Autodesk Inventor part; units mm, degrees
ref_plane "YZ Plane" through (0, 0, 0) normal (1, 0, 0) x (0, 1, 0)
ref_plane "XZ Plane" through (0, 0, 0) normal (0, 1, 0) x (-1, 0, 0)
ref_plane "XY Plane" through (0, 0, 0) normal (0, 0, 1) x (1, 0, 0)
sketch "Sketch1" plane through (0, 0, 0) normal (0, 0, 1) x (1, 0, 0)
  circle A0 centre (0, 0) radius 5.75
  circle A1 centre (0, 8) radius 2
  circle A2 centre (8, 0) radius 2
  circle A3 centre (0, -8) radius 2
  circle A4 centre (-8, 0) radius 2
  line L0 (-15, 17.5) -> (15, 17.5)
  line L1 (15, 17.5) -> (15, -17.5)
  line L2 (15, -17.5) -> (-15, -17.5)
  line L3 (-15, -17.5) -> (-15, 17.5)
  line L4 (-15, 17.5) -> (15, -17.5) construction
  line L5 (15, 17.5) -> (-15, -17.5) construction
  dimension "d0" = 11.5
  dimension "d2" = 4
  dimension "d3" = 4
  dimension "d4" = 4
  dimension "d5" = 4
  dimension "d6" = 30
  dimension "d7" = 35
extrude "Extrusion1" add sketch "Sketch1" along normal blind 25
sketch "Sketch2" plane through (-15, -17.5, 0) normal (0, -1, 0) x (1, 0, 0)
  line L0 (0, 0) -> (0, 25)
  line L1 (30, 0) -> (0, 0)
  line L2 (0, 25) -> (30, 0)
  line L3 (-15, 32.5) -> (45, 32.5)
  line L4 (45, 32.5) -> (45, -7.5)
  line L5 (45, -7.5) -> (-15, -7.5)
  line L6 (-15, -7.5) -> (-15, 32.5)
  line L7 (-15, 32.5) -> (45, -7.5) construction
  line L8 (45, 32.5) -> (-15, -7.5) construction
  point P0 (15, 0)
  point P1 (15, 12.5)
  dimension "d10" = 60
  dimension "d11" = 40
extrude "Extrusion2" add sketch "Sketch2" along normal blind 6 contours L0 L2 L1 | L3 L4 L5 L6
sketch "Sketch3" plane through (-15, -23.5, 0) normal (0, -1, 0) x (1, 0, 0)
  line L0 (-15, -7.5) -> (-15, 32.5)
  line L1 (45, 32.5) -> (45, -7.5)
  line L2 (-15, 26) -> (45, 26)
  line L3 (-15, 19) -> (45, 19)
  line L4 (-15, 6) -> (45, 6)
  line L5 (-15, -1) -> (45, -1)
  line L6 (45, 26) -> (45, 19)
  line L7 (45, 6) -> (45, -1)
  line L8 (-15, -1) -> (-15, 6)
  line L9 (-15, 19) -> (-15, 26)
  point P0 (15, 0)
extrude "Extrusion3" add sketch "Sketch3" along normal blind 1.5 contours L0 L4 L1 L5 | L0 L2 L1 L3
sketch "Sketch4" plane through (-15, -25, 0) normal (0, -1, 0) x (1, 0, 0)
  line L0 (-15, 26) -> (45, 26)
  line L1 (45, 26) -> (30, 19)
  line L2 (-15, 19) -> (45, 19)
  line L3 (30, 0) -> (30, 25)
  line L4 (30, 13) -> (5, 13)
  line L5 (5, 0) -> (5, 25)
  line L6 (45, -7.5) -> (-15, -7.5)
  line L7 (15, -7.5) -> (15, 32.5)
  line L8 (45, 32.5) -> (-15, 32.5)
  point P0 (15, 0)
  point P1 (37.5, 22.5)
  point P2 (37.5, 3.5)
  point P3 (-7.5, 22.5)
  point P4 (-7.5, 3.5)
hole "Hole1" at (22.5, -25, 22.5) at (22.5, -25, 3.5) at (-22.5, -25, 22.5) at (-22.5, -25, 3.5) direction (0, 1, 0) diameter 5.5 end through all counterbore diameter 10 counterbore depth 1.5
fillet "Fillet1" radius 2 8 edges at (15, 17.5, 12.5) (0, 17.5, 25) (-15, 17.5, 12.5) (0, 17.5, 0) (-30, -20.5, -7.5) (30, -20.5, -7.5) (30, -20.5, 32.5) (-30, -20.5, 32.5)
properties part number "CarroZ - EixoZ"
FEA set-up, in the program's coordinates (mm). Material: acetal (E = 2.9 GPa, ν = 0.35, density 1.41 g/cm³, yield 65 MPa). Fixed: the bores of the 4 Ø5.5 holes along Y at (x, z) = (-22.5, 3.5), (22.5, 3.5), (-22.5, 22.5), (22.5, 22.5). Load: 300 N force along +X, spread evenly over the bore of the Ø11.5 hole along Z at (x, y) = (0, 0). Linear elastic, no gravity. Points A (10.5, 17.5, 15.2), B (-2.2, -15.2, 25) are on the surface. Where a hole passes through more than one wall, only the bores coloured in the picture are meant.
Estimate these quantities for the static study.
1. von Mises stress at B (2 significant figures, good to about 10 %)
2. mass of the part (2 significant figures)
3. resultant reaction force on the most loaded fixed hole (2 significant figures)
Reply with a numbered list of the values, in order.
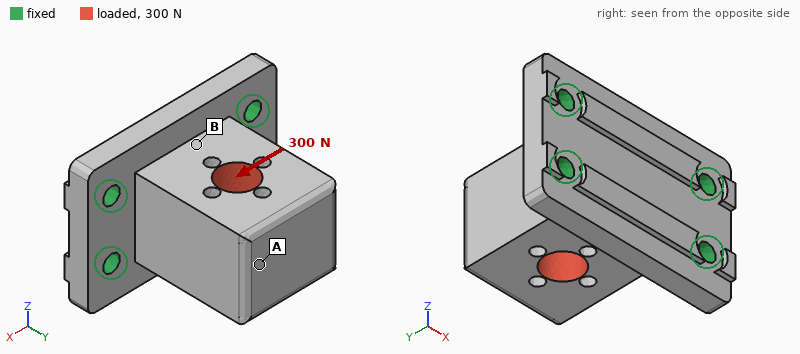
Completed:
1. 0.95 MPa
2. 52 g
3. 120 N
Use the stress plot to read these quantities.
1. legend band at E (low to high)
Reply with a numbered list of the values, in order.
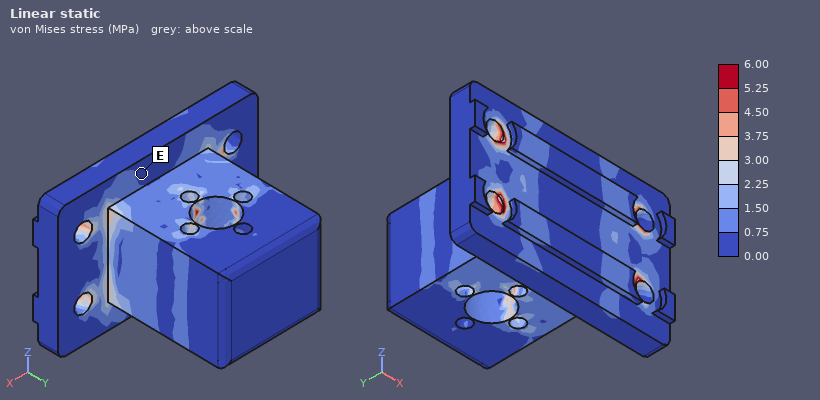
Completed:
1. 0.00 to 0.75 MPa
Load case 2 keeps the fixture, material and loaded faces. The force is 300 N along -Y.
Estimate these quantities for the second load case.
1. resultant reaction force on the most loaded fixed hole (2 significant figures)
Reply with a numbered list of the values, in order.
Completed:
1. 83 N
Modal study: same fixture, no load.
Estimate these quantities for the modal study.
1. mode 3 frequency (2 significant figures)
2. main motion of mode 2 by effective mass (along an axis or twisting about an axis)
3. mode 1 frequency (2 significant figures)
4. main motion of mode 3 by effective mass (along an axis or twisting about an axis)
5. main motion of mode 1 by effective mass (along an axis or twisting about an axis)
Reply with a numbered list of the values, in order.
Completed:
1. 3300 Hz
2. along X
3. 1500 Hz
4. along Y
5. along Z
